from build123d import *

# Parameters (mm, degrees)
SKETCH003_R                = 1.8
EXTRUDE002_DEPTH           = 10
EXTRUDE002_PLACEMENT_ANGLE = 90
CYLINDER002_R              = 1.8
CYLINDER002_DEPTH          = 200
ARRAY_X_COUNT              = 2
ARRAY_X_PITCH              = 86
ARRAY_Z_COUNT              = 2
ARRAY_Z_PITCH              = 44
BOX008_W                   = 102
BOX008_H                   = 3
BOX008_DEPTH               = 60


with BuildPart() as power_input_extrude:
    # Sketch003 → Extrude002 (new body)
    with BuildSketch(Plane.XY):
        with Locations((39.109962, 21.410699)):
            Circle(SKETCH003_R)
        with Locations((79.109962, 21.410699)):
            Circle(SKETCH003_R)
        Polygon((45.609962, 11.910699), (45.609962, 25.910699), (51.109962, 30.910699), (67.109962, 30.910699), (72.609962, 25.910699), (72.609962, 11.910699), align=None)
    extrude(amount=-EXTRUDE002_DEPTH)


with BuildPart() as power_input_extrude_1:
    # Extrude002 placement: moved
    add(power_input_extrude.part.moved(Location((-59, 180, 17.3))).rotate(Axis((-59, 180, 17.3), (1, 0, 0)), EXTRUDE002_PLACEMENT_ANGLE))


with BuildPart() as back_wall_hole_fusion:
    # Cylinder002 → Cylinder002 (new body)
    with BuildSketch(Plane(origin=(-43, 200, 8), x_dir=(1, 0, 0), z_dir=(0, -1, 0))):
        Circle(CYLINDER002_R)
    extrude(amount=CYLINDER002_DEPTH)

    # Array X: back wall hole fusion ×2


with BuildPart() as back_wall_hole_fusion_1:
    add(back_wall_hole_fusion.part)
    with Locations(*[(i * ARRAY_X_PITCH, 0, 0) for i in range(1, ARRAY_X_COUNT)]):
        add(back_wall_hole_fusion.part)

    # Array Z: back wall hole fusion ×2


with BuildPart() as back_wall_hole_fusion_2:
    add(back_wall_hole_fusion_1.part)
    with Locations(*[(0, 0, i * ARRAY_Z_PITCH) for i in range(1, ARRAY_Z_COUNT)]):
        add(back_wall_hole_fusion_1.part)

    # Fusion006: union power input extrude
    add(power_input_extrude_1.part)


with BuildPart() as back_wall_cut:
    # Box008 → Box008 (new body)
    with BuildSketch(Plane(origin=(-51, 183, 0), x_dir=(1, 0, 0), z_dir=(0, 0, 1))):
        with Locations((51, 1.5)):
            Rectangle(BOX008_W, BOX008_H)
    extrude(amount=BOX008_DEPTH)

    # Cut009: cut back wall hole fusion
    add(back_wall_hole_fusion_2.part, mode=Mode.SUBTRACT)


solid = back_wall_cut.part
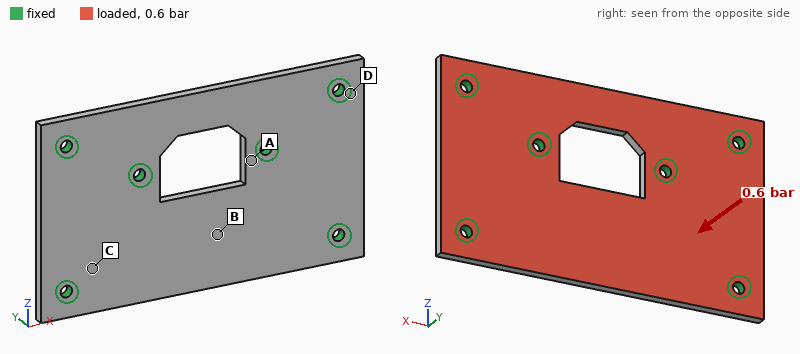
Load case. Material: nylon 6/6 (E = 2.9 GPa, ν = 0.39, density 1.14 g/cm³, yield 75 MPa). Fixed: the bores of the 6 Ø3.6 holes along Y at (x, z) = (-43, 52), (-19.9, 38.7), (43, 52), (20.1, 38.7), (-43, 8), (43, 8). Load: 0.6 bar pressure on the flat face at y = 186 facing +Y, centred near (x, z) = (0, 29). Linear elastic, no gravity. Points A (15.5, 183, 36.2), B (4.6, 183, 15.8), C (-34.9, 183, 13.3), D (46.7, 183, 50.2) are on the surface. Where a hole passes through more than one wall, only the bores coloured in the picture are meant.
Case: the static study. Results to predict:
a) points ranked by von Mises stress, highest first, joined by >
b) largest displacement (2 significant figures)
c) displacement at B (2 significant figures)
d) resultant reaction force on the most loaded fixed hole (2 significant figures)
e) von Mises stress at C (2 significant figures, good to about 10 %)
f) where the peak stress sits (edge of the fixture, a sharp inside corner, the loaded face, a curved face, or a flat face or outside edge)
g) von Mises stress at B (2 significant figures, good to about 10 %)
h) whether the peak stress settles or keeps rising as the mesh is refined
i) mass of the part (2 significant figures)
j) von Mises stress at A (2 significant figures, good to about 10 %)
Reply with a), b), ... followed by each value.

a) A > C > B > D
b) 0.96 mm
c) 0.54 mm
d) 77 N
e) 7.3 MPa
f) edge of the fixture
g) 5.3 MPa
h) keeps rising
i) 19 g
j) 12 MPa
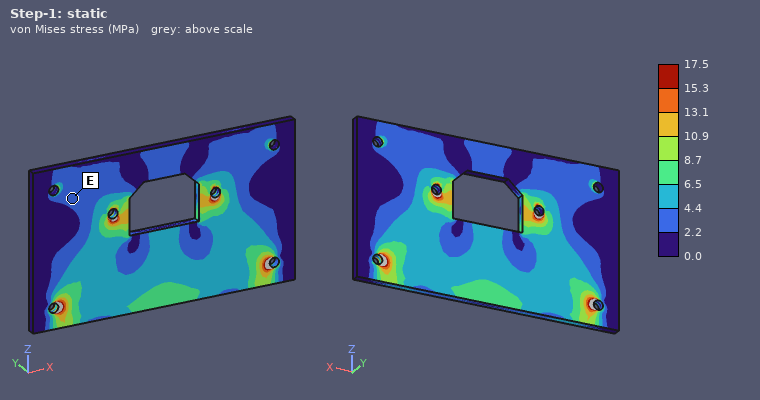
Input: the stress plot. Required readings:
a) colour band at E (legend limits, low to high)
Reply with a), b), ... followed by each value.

a) 2.2 to 4.4 MPa
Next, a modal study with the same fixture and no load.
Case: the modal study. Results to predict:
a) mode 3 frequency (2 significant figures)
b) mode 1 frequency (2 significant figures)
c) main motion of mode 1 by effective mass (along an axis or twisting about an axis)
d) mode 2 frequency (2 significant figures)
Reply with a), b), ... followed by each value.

a) 2100 Hz
b) 910 Hz
c) along Y
d) 1500 Hz
